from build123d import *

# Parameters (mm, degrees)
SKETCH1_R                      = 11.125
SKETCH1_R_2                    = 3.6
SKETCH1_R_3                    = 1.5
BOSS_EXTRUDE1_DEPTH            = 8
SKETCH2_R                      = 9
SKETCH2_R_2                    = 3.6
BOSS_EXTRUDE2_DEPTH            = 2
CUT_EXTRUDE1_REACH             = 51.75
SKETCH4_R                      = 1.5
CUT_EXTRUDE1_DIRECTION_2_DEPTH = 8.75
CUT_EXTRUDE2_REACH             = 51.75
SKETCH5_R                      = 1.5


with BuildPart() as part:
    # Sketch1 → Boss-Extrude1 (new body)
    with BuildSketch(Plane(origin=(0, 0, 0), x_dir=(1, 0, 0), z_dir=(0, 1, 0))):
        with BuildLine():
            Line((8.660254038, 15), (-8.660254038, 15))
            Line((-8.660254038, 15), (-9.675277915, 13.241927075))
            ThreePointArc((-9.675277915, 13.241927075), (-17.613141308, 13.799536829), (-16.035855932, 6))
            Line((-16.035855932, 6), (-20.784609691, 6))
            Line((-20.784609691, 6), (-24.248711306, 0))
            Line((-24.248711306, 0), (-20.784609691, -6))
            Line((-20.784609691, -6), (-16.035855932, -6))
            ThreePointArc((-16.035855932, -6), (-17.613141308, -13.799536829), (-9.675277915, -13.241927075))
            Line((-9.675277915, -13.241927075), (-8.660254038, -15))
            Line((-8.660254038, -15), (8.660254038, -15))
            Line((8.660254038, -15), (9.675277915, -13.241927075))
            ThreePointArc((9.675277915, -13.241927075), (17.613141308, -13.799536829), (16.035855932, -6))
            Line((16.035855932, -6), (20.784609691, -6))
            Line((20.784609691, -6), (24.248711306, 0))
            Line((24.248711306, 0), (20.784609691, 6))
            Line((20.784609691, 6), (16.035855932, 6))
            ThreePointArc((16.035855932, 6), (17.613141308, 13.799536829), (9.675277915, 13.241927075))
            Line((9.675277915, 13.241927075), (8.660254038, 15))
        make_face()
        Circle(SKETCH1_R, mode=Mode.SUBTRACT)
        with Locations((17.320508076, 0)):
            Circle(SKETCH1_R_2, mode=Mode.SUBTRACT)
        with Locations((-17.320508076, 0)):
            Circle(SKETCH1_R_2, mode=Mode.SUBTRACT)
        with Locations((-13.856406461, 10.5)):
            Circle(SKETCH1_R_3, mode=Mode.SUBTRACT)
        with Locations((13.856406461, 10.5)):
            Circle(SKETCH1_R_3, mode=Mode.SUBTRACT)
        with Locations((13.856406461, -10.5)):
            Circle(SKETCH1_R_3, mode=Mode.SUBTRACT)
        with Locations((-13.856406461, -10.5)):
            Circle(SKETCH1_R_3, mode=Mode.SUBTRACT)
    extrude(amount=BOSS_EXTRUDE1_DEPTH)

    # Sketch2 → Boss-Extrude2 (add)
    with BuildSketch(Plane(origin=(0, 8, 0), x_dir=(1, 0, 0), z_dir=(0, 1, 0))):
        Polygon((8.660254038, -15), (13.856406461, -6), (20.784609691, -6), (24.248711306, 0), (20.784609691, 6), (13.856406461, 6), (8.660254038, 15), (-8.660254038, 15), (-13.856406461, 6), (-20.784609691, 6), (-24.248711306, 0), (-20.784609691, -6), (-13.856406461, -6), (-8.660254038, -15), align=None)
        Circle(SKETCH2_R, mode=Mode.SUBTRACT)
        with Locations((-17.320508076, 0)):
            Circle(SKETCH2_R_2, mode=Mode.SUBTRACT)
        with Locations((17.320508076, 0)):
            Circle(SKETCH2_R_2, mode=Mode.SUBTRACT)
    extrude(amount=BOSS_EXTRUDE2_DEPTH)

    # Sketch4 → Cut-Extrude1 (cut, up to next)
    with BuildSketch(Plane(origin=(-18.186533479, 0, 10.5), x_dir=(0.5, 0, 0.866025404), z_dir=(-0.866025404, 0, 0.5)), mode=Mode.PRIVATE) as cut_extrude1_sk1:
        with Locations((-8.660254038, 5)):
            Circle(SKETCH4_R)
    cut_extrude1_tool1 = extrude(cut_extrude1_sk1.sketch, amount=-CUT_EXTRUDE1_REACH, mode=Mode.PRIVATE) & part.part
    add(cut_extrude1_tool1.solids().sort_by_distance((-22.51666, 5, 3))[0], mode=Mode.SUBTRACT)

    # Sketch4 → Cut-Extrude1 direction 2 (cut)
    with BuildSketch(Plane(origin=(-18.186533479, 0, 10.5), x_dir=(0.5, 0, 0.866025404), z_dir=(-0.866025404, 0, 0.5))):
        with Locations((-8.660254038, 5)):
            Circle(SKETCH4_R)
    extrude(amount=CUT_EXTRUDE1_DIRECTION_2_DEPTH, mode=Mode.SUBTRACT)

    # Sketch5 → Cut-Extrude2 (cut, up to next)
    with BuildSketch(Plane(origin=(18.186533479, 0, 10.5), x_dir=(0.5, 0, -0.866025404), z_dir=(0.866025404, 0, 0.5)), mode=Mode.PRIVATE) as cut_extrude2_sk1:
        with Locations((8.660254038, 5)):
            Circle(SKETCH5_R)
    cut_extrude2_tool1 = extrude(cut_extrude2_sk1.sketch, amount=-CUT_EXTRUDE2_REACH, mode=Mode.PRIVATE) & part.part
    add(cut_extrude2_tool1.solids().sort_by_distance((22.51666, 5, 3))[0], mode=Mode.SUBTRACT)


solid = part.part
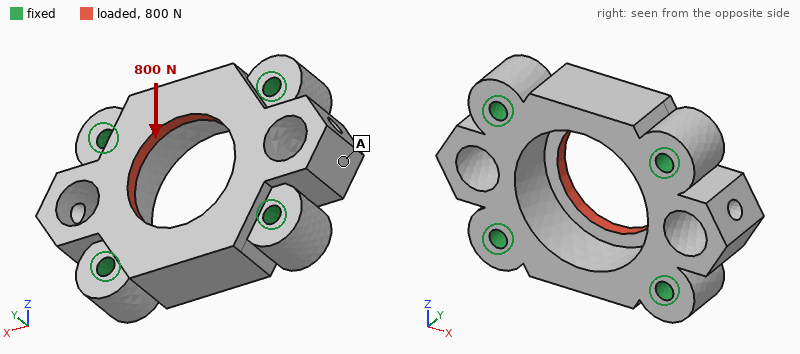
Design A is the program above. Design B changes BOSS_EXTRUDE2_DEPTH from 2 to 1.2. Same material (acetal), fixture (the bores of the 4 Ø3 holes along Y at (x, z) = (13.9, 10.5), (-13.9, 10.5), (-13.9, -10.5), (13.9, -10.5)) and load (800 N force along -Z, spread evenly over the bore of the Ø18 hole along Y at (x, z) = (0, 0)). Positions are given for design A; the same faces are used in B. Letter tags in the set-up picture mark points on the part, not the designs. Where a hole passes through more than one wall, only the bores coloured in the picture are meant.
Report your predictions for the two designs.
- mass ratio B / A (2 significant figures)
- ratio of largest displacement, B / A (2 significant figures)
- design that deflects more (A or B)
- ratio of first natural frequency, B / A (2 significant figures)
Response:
0.93
1.2
B
1.0
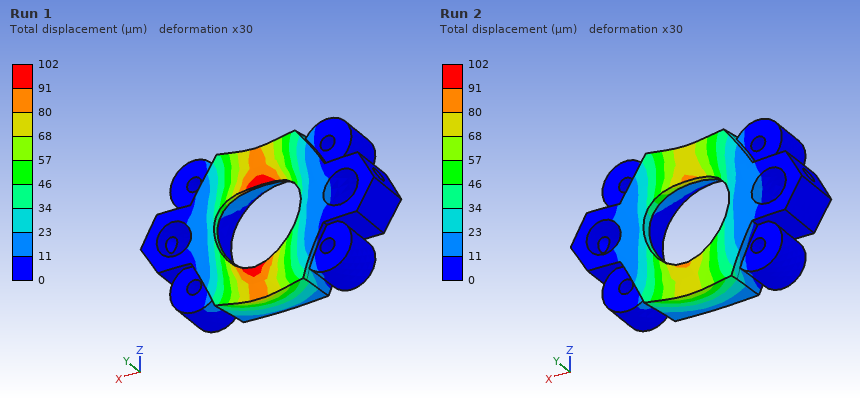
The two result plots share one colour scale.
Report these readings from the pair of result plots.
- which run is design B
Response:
Run 1
